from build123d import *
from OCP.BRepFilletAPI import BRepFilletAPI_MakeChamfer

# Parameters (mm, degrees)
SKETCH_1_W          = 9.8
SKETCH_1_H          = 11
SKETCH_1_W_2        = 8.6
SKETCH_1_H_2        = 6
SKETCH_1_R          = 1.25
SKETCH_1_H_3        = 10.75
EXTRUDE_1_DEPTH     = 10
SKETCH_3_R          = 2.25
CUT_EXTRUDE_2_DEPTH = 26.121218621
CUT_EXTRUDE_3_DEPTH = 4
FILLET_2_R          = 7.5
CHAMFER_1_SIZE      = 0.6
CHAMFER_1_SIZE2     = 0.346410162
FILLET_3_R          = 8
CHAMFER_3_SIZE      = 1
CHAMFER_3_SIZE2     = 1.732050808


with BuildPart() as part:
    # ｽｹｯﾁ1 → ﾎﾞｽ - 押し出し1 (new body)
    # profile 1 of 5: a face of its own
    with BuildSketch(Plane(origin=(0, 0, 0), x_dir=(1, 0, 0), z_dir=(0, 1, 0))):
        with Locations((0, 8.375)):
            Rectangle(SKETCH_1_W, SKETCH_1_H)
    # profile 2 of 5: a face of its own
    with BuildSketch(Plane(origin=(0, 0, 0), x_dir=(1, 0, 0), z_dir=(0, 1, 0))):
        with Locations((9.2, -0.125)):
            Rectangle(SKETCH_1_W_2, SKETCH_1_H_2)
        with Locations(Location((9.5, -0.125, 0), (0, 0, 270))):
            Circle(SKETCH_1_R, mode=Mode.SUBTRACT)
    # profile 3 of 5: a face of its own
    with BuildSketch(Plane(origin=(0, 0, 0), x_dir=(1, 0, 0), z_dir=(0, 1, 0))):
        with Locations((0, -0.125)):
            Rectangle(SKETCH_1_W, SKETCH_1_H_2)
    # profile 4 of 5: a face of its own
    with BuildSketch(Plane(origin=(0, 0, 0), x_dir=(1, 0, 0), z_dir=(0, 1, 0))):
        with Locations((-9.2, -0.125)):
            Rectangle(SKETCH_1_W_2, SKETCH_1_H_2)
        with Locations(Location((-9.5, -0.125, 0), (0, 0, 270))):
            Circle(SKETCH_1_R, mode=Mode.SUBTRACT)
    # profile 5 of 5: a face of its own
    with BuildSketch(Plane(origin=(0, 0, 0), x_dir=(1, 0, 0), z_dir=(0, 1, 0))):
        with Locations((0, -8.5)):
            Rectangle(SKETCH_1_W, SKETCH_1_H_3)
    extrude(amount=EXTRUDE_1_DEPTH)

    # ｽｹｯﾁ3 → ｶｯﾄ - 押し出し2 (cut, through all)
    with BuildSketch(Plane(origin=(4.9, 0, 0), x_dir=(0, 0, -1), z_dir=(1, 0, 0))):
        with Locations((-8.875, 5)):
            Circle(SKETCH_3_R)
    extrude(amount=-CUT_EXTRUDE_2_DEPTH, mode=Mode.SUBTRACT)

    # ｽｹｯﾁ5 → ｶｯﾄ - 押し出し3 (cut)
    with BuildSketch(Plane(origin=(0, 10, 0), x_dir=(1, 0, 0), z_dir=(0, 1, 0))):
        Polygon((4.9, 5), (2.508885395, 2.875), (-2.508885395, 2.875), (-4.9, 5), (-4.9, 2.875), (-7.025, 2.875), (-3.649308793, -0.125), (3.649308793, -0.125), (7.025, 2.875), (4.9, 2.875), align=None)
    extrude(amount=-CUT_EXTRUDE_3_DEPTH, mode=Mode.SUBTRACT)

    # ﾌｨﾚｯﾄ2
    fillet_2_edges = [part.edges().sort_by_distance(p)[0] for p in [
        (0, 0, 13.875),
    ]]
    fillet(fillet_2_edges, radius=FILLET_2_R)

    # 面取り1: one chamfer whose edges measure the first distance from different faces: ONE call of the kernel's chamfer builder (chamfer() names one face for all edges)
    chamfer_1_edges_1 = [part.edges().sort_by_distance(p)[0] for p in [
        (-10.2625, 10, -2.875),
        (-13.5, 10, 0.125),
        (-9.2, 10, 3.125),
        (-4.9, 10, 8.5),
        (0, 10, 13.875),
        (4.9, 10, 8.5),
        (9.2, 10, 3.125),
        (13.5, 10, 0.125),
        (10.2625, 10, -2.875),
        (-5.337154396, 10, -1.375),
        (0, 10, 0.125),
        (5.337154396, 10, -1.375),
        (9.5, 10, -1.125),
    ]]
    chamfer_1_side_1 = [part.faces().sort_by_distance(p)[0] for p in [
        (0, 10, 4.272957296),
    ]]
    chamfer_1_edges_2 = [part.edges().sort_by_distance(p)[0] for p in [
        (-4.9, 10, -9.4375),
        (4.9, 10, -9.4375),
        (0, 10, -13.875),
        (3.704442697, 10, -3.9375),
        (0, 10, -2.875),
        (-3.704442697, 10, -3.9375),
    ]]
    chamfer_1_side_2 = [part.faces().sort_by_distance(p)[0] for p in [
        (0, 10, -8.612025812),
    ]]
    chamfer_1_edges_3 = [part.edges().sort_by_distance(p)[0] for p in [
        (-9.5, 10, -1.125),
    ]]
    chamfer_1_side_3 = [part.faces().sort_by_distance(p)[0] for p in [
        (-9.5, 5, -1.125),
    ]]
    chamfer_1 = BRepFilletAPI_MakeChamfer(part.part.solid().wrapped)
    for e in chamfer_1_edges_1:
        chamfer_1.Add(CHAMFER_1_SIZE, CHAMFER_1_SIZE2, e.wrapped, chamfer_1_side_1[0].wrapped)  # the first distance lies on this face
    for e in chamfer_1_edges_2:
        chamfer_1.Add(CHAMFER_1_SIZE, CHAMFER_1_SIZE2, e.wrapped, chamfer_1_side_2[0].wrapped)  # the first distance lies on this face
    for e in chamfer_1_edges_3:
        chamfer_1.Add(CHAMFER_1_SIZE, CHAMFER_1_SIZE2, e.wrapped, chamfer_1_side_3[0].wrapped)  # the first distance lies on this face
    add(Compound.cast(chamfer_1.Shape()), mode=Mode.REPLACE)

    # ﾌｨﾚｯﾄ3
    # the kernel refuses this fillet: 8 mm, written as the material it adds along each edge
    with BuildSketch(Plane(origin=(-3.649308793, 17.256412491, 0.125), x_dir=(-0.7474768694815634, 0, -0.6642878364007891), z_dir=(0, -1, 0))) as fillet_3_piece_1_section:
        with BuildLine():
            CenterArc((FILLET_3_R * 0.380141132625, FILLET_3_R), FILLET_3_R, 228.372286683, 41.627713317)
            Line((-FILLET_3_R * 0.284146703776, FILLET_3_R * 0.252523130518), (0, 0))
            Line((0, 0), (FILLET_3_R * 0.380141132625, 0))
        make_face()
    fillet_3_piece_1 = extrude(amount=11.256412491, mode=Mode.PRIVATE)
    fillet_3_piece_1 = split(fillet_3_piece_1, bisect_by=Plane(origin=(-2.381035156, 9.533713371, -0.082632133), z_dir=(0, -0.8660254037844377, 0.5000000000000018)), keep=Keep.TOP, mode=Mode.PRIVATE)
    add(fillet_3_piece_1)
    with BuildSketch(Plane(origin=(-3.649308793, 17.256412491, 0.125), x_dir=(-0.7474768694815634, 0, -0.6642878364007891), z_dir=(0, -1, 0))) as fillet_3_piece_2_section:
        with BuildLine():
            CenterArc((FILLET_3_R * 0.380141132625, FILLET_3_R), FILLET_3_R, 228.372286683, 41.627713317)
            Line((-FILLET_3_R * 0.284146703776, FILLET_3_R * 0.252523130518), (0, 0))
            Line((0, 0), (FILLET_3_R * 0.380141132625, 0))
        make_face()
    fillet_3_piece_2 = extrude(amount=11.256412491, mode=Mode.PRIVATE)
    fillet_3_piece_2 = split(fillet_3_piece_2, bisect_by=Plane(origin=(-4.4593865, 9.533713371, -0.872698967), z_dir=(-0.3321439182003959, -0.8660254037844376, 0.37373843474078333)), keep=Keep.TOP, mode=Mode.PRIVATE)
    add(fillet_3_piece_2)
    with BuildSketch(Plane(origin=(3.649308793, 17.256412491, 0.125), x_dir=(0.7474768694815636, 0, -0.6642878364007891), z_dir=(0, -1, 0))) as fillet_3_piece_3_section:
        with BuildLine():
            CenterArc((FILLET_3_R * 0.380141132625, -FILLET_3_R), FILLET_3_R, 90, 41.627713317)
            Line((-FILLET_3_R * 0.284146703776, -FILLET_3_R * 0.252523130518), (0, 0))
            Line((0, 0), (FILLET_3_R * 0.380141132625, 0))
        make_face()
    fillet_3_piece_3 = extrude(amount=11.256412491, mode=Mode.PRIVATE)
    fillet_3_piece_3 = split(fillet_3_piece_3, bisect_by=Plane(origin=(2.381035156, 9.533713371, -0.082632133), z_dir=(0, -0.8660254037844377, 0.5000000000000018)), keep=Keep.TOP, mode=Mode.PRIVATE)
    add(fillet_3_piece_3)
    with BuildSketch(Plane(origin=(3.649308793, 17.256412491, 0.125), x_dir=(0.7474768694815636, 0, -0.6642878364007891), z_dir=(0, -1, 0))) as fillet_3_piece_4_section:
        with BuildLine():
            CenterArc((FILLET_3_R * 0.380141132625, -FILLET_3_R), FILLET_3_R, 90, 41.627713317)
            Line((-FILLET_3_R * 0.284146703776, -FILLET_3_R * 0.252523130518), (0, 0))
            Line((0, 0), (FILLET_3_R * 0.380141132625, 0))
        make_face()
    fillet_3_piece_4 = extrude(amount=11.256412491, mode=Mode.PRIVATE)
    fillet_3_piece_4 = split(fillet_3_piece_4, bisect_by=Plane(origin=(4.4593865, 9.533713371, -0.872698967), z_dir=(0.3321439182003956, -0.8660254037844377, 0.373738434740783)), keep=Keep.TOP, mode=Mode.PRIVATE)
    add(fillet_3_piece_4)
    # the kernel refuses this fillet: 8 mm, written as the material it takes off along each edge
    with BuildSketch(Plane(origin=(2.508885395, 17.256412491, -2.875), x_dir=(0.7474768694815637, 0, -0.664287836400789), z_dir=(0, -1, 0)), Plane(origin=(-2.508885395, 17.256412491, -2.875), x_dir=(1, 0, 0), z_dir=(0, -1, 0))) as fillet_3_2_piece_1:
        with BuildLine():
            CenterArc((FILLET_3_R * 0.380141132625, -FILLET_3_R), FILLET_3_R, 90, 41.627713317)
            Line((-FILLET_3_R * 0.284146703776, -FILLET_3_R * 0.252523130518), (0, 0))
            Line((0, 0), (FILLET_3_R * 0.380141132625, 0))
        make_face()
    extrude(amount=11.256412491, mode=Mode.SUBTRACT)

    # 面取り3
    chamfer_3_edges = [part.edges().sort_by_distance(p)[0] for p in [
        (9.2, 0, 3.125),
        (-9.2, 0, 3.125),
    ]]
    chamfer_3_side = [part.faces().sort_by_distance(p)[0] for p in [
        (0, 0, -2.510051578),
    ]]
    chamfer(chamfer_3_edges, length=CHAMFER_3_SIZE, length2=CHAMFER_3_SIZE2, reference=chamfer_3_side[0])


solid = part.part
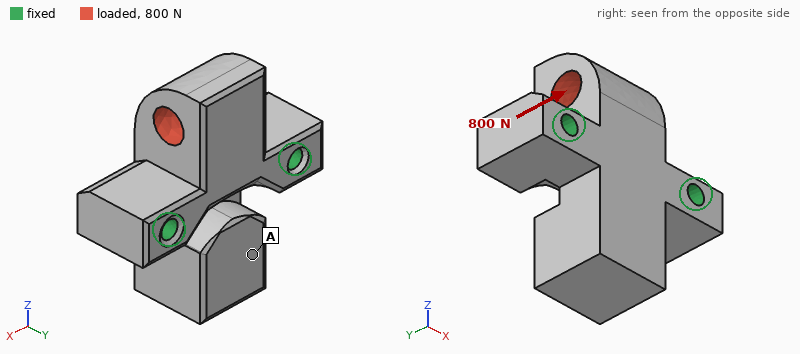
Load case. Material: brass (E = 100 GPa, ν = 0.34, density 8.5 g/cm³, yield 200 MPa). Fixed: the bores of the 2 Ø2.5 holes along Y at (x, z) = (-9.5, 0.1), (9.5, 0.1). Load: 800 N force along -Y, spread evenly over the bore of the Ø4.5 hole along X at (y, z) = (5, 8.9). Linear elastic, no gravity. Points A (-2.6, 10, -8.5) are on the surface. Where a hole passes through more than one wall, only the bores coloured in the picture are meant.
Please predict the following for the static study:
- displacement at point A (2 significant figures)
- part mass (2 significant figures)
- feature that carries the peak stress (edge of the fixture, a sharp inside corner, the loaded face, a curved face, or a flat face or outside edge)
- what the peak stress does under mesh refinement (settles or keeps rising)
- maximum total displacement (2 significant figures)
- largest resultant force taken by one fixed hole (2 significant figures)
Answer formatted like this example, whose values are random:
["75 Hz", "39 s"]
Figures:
["7.5 µm", "27 g", "edge of the fixture", "keeps rising", "23 µm", "430 N"]
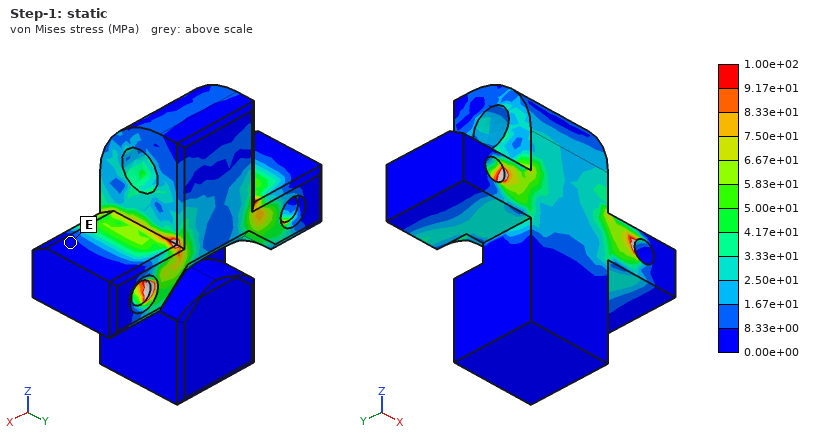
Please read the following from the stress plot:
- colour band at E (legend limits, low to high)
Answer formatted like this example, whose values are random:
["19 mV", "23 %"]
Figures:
["0.00e+00 to 8.33e+00 MPa"]
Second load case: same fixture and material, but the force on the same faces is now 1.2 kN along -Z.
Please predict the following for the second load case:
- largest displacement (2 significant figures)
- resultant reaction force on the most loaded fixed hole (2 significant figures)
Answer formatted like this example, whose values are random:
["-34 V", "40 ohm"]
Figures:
["4.8 µm", "640 N"]
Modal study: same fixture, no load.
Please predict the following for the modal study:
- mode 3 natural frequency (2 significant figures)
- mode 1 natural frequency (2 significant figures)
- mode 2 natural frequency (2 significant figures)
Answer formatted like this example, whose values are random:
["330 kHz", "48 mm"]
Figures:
["16 kHz", "8700 Hz", "16 kHz"]
